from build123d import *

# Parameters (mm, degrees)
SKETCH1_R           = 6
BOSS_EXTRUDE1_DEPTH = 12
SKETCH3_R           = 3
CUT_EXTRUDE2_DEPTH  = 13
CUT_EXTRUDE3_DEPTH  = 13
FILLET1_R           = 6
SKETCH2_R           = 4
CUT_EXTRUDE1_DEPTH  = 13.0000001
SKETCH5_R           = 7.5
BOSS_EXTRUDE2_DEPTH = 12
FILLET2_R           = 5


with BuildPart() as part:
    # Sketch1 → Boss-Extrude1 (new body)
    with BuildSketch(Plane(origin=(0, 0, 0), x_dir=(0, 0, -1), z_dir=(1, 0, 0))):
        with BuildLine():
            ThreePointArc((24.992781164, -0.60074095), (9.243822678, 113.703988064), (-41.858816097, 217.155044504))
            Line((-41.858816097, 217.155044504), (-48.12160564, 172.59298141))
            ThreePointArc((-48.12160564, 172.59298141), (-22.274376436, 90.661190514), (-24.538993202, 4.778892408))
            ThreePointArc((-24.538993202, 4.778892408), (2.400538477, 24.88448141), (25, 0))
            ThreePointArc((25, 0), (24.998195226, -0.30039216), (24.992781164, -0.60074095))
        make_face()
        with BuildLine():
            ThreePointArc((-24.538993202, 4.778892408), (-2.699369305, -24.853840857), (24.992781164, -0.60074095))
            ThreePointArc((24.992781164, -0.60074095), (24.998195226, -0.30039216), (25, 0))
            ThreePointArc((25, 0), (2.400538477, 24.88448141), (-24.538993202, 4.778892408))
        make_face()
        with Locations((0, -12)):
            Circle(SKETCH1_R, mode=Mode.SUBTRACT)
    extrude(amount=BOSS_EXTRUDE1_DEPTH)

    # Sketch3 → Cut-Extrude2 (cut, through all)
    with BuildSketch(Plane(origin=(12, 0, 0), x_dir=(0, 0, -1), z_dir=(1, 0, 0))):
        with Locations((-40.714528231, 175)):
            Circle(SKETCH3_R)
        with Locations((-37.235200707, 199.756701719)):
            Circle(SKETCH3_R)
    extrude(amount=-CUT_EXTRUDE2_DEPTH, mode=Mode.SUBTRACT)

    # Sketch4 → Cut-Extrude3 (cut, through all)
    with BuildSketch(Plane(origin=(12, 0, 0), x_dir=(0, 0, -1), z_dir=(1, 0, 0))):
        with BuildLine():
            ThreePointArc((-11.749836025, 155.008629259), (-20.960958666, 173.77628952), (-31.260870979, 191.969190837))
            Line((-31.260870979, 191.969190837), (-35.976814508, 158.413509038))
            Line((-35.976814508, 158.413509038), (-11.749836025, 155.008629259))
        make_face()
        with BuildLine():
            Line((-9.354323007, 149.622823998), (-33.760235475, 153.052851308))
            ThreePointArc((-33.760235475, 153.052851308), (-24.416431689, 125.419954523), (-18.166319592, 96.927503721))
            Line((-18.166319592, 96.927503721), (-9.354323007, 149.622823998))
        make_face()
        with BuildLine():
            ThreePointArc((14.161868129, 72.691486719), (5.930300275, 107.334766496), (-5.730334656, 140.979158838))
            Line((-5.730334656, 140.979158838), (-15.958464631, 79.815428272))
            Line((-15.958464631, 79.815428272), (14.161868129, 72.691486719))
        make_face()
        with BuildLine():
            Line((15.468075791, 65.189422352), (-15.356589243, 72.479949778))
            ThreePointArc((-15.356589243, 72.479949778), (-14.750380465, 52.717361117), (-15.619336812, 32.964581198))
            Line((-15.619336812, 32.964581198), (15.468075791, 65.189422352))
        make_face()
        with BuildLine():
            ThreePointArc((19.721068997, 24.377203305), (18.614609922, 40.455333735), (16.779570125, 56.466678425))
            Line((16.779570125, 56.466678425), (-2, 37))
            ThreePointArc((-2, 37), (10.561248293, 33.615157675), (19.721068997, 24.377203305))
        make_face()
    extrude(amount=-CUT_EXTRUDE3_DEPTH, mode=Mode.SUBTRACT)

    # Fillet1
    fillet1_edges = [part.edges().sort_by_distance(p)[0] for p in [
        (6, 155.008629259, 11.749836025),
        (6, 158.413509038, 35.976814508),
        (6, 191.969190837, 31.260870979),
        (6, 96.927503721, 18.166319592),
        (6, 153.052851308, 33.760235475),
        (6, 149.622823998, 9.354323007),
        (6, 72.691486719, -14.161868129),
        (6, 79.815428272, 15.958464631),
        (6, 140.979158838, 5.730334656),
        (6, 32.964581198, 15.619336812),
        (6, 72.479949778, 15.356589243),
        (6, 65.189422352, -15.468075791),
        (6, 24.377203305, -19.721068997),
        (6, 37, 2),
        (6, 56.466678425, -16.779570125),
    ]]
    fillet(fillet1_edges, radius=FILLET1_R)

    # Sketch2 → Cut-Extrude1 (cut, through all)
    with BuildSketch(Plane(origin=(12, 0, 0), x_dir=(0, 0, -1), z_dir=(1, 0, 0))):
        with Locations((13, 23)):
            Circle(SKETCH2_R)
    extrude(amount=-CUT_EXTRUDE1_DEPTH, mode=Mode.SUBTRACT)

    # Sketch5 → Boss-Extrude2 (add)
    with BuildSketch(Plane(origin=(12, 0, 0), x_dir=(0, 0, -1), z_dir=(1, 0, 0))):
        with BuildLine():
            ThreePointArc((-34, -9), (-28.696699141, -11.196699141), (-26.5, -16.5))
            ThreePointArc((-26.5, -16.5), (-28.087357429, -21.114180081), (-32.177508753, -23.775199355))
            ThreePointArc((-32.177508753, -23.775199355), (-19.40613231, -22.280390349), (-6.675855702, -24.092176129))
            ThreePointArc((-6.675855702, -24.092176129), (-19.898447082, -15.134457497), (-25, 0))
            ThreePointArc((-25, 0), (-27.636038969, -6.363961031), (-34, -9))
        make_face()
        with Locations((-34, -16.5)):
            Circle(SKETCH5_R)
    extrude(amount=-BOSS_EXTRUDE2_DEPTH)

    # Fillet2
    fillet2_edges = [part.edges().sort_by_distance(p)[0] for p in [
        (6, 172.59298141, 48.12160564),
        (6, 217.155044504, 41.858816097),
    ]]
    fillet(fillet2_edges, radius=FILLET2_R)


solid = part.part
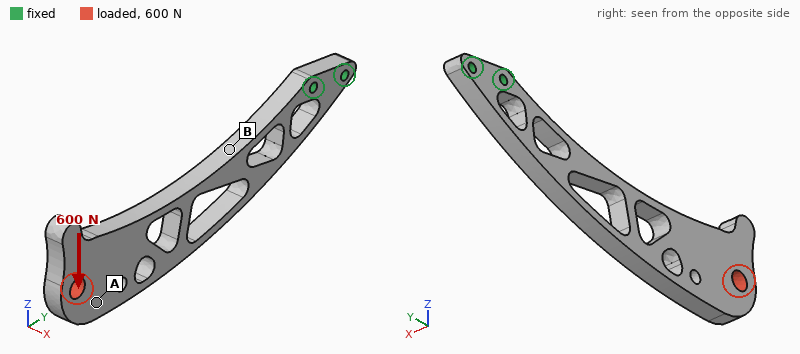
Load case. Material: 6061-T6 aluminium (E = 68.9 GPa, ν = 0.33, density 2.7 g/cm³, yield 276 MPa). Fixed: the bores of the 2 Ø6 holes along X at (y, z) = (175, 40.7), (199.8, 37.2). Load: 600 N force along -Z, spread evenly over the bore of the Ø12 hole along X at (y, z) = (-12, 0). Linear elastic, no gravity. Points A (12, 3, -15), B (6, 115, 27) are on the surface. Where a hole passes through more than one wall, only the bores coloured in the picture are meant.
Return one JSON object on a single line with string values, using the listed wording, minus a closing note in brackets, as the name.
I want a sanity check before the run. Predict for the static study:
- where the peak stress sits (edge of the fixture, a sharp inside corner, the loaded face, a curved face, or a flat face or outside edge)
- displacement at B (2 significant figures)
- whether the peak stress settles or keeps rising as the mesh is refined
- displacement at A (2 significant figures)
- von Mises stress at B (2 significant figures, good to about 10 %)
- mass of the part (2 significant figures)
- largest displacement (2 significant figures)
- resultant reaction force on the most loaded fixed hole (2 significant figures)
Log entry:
{"where the peak stress sits": "edge of the fixture", "displacement at B": "0.23 mm", "whether the peak stress settles or keeps rising as the mesh is refined": "keeps rising", "displacement at A": "1.1 mm", "von Mises stress at B": "64 MPa", "mass of the part": "200 g", "largest displacement": "1.2 mm", "resultant reaction force on the most loaded fixed hole": "4.7 kN"}
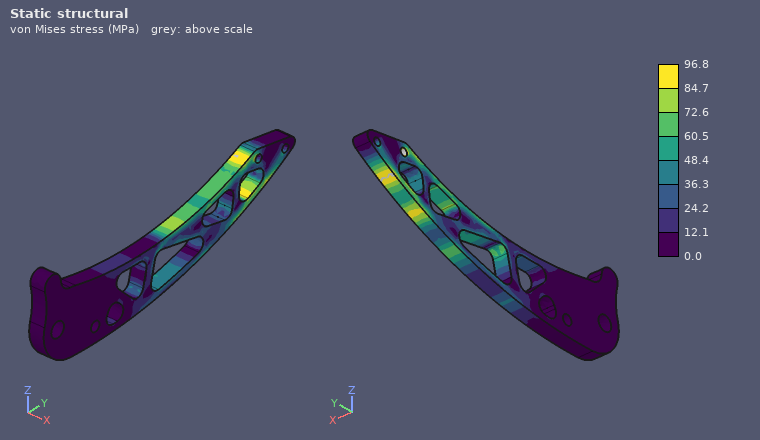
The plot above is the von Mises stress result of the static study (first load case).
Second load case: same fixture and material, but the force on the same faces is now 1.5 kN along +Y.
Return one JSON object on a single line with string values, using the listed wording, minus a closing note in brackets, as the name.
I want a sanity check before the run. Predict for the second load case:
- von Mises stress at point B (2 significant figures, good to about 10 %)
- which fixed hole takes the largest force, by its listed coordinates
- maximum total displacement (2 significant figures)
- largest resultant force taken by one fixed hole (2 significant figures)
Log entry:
{"von Mises stress at point B": "5.5 MPa", "which fixed hole takes the largest force, by its listed coordinates": "(199.8, 37.2)", "maximum total displacement": "0.44 mm", "largest resultant force taken by one fixed hole": "2.4 kN"}
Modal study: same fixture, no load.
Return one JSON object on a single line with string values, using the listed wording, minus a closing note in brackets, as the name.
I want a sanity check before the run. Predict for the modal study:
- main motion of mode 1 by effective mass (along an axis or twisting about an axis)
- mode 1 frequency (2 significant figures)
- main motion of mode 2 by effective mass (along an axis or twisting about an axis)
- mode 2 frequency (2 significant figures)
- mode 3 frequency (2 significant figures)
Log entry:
{"main motion of mode 1 by effective mass": "along X", "mode 1 frequency": "140 Hz", "main motion of mode 2 by effective mass": "along Z", "mode 2 frequency": "380 Hz", "mode 3 frequency": "680 Hz"}
